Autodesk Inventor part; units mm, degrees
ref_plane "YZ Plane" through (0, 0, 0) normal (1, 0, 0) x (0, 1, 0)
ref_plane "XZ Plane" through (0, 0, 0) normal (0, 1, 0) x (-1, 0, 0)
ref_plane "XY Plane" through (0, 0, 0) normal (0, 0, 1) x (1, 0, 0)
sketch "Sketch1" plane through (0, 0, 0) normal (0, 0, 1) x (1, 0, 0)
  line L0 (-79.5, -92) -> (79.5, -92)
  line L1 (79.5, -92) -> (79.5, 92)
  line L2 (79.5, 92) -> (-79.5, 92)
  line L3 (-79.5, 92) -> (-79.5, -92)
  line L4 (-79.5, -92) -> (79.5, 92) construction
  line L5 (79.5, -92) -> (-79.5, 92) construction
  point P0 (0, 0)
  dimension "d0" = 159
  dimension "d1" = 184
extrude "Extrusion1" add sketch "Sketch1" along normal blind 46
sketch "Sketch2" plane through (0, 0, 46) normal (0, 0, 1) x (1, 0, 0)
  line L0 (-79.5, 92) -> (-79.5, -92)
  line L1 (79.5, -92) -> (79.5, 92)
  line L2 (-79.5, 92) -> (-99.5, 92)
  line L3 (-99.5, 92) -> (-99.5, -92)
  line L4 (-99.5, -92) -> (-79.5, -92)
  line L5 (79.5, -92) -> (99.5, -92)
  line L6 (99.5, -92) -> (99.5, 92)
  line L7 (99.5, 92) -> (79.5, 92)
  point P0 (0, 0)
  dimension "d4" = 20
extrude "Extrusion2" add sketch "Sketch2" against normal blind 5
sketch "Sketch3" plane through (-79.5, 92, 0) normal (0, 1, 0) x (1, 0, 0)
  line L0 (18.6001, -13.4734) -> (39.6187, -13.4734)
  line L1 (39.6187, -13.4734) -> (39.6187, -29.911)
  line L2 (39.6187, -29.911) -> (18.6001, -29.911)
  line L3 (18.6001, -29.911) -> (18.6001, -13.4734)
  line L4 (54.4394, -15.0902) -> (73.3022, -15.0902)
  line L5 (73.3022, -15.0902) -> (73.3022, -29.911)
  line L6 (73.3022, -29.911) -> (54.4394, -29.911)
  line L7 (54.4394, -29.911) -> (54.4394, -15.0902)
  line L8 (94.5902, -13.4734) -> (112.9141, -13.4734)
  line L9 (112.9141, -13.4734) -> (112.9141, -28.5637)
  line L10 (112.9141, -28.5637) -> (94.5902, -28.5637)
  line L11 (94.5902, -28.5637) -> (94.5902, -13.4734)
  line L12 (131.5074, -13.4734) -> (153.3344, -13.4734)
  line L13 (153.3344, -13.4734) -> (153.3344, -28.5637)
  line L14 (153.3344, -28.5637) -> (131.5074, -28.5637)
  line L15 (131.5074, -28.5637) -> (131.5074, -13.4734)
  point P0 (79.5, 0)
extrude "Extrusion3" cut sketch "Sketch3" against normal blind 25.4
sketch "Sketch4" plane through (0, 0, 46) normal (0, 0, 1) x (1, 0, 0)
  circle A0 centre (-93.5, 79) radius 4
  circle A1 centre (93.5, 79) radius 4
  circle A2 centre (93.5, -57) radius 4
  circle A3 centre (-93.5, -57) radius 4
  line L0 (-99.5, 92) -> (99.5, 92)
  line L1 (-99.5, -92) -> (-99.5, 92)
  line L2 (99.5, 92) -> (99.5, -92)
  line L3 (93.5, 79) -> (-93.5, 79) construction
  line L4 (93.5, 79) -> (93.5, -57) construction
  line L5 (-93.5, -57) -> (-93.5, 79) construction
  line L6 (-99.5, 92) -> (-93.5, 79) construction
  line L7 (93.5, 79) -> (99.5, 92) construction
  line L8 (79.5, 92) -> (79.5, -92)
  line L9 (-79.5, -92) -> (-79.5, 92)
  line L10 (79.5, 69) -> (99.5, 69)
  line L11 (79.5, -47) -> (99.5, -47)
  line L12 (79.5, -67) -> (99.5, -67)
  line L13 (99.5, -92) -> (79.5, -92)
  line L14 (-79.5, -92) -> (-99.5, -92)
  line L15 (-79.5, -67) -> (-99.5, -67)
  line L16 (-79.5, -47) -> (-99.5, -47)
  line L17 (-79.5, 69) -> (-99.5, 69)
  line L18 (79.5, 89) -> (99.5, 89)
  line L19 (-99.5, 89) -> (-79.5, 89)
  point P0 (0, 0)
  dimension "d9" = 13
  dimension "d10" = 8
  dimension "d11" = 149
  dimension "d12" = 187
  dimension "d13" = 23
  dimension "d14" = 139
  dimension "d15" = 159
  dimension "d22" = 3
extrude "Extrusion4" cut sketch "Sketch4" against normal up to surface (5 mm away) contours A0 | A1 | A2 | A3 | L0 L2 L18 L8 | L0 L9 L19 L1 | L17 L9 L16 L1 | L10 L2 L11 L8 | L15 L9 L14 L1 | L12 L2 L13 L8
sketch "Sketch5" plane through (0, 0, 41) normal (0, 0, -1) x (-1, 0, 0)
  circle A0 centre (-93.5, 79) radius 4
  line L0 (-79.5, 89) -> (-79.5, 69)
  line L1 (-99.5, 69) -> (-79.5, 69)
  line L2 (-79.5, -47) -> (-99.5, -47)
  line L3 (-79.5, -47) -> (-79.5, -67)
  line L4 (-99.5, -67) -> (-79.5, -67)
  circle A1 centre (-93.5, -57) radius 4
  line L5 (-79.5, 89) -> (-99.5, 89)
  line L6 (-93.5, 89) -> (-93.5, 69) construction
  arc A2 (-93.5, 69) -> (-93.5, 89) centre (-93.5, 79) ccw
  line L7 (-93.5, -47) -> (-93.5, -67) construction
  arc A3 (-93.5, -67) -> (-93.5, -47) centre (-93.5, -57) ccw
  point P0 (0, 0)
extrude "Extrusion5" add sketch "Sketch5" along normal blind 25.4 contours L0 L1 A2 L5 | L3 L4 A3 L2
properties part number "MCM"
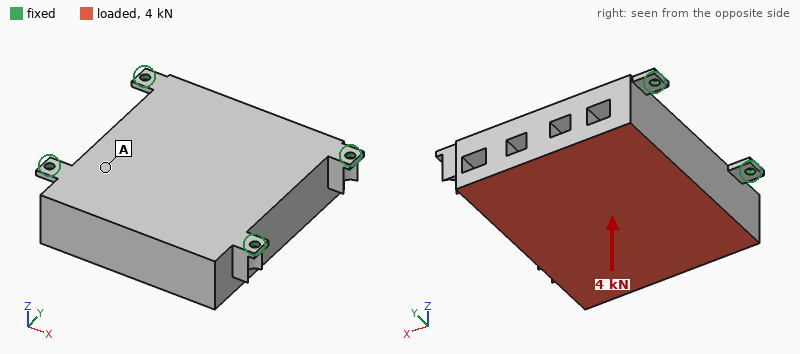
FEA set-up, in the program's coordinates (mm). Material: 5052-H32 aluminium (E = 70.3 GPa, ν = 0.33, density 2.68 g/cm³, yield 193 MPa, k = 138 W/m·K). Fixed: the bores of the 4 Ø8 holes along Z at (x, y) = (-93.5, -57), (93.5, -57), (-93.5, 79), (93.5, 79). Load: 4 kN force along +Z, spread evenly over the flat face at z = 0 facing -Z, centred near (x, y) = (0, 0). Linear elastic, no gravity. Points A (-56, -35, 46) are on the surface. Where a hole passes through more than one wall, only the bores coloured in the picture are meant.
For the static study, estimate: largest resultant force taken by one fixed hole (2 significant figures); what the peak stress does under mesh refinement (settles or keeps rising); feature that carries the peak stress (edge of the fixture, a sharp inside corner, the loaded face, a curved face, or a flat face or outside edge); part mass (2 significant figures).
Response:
1.4 kN
keeps rising
edge of the fixture
3.6 kg
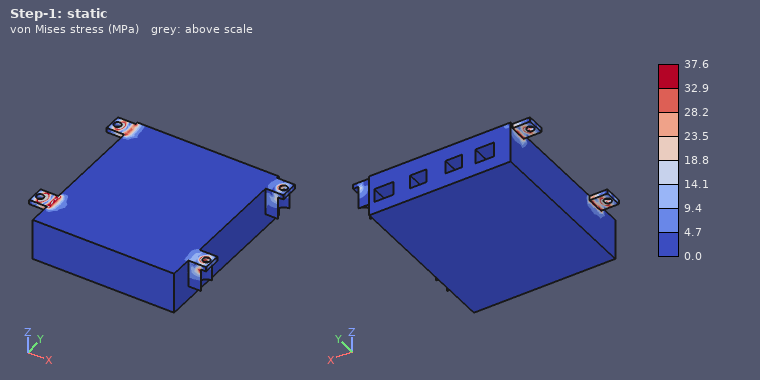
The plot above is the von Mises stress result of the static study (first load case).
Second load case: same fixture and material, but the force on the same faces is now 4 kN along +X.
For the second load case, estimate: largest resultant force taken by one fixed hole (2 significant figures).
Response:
1.3 kN
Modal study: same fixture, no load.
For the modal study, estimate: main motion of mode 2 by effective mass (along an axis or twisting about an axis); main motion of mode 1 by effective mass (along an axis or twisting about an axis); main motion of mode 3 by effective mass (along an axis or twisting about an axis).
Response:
along Y
along Z
along Y
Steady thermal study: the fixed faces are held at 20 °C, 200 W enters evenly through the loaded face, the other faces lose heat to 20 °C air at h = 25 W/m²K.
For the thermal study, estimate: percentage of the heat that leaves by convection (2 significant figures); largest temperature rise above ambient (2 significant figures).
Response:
33 %
41 K
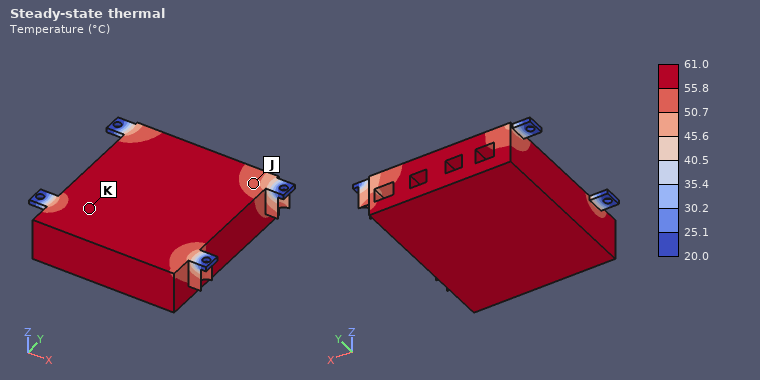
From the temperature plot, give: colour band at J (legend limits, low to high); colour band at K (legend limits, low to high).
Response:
50.7 to 55.8 °C
55.8 to 61.0 °C
